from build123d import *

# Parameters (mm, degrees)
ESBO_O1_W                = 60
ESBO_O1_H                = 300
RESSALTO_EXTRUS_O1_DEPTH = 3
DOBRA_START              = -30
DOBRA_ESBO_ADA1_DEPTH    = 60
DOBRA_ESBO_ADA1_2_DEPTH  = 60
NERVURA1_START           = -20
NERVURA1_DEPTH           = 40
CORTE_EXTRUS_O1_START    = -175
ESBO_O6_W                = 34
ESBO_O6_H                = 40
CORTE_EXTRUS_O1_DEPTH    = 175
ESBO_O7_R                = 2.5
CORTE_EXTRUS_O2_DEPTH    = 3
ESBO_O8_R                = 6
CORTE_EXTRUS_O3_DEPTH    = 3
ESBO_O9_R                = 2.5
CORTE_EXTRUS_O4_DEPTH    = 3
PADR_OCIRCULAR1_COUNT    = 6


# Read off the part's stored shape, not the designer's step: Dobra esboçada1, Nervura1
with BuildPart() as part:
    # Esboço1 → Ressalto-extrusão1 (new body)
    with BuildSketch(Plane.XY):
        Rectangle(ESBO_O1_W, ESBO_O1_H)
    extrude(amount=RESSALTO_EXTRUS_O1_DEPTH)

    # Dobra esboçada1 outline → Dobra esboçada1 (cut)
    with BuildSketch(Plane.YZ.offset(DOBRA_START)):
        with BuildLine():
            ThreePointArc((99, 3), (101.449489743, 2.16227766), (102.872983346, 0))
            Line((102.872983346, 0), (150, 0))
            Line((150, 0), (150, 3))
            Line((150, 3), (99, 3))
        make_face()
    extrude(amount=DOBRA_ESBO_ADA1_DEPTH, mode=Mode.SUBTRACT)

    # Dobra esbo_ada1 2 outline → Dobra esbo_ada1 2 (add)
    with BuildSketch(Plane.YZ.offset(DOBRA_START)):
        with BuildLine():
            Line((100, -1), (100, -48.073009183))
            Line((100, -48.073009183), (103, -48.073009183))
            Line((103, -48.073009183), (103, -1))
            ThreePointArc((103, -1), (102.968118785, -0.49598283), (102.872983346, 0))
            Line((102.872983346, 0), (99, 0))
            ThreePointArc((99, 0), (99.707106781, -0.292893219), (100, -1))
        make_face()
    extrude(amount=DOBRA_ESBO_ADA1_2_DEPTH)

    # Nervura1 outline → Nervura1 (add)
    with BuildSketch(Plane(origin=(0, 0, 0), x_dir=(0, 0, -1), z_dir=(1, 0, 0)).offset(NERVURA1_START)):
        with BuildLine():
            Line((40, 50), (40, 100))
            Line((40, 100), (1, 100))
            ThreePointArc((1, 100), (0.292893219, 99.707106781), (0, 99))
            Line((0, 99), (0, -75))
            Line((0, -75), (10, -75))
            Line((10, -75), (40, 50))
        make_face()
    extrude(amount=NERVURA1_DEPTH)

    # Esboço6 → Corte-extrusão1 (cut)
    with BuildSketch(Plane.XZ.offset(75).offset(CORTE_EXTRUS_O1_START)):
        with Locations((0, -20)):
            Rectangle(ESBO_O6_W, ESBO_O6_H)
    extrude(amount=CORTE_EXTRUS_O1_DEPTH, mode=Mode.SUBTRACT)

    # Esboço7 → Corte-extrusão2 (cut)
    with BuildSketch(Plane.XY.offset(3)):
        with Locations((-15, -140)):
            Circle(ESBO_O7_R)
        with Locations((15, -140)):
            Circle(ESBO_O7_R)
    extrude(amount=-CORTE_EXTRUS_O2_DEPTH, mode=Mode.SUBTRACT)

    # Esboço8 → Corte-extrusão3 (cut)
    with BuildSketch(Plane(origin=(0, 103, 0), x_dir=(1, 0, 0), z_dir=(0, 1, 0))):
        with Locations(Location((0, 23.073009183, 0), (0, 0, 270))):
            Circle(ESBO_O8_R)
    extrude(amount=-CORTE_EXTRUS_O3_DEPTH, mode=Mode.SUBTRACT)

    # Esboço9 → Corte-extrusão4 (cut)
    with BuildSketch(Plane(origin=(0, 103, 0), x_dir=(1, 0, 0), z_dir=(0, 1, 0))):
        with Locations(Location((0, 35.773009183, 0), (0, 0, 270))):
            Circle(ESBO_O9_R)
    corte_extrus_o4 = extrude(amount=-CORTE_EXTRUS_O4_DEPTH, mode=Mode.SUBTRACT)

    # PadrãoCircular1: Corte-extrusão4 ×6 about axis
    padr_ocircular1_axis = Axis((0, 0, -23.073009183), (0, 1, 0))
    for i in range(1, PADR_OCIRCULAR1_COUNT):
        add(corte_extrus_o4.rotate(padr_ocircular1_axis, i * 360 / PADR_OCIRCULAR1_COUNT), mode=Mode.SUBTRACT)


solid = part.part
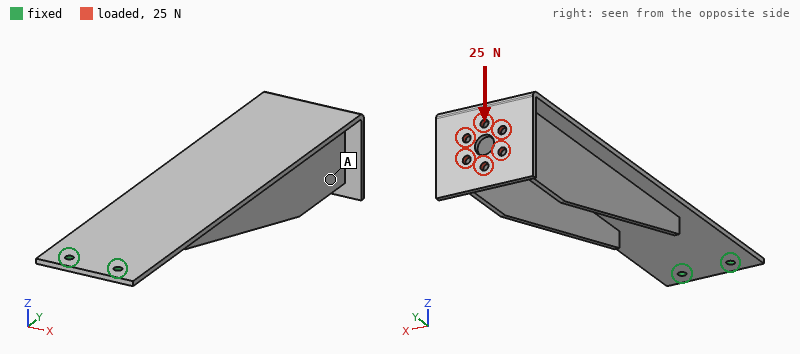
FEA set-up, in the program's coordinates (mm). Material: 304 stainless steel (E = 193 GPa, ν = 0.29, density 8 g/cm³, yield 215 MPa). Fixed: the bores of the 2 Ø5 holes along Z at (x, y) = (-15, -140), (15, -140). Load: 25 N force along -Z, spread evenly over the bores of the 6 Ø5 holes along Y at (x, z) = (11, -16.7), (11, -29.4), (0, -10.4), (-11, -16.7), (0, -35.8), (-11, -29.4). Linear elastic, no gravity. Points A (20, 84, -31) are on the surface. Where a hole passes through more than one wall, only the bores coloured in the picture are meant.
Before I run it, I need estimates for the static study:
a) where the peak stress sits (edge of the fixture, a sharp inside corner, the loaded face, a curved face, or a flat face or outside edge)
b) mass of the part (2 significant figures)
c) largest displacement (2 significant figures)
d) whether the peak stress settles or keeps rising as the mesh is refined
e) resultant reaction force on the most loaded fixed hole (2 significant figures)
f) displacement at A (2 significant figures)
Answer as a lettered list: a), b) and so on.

a) edge of the fixture
b) 670 g
c) 2.9 mm
d) keeps rising
e) 13 N
f) 2.6 mm
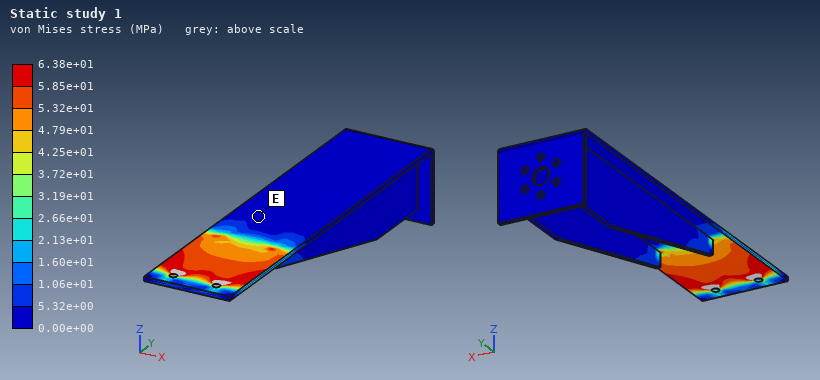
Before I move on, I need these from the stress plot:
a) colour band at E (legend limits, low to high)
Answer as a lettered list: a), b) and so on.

a) 0.00e+00 to 5.32e+00 MPa
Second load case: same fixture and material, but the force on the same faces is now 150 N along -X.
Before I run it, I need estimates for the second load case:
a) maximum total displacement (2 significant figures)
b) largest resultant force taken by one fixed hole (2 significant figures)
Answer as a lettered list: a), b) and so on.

a) 0.66 mm
b) 1.1 kN
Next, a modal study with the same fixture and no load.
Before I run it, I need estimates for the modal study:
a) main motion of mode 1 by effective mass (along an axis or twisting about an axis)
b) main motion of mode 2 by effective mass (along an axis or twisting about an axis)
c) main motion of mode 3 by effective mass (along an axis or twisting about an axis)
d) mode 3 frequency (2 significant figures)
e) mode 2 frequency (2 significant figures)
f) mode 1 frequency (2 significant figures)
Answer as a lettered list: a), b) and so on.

a) along Z
b) along X
c) along Z
d) 470 Hz
e) 180 Hz
f) 28 Hz
